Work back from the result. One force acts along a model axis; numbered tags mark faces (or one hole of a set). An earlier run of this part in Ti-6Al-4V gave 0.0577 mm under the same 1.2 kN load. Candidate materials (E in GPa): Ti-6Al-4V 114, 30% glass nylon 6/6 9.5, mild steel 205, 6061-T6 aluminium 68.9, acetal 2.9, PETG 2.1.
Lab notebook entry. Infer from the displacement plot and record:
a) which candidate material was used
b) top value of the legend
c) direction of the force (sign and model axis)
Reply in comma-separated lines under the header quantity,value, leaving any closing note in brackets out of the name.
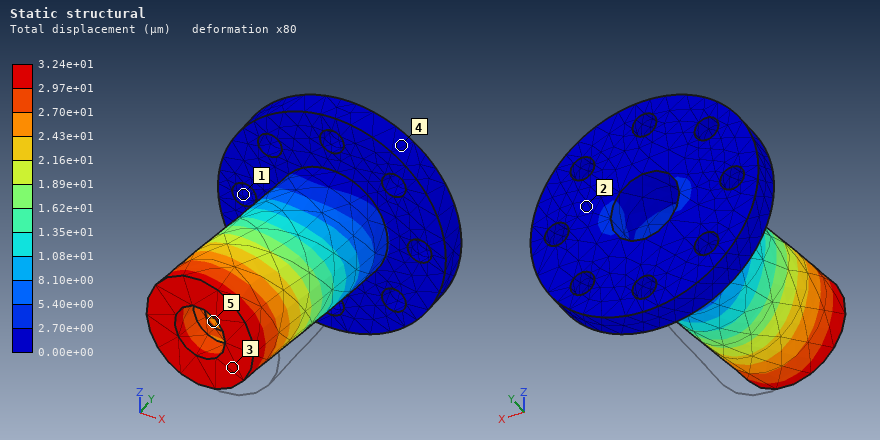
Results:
quantity,value
which candidate material was used,mild steel
top value of the legend,3.24e+01 µm
direction of the force,-X
